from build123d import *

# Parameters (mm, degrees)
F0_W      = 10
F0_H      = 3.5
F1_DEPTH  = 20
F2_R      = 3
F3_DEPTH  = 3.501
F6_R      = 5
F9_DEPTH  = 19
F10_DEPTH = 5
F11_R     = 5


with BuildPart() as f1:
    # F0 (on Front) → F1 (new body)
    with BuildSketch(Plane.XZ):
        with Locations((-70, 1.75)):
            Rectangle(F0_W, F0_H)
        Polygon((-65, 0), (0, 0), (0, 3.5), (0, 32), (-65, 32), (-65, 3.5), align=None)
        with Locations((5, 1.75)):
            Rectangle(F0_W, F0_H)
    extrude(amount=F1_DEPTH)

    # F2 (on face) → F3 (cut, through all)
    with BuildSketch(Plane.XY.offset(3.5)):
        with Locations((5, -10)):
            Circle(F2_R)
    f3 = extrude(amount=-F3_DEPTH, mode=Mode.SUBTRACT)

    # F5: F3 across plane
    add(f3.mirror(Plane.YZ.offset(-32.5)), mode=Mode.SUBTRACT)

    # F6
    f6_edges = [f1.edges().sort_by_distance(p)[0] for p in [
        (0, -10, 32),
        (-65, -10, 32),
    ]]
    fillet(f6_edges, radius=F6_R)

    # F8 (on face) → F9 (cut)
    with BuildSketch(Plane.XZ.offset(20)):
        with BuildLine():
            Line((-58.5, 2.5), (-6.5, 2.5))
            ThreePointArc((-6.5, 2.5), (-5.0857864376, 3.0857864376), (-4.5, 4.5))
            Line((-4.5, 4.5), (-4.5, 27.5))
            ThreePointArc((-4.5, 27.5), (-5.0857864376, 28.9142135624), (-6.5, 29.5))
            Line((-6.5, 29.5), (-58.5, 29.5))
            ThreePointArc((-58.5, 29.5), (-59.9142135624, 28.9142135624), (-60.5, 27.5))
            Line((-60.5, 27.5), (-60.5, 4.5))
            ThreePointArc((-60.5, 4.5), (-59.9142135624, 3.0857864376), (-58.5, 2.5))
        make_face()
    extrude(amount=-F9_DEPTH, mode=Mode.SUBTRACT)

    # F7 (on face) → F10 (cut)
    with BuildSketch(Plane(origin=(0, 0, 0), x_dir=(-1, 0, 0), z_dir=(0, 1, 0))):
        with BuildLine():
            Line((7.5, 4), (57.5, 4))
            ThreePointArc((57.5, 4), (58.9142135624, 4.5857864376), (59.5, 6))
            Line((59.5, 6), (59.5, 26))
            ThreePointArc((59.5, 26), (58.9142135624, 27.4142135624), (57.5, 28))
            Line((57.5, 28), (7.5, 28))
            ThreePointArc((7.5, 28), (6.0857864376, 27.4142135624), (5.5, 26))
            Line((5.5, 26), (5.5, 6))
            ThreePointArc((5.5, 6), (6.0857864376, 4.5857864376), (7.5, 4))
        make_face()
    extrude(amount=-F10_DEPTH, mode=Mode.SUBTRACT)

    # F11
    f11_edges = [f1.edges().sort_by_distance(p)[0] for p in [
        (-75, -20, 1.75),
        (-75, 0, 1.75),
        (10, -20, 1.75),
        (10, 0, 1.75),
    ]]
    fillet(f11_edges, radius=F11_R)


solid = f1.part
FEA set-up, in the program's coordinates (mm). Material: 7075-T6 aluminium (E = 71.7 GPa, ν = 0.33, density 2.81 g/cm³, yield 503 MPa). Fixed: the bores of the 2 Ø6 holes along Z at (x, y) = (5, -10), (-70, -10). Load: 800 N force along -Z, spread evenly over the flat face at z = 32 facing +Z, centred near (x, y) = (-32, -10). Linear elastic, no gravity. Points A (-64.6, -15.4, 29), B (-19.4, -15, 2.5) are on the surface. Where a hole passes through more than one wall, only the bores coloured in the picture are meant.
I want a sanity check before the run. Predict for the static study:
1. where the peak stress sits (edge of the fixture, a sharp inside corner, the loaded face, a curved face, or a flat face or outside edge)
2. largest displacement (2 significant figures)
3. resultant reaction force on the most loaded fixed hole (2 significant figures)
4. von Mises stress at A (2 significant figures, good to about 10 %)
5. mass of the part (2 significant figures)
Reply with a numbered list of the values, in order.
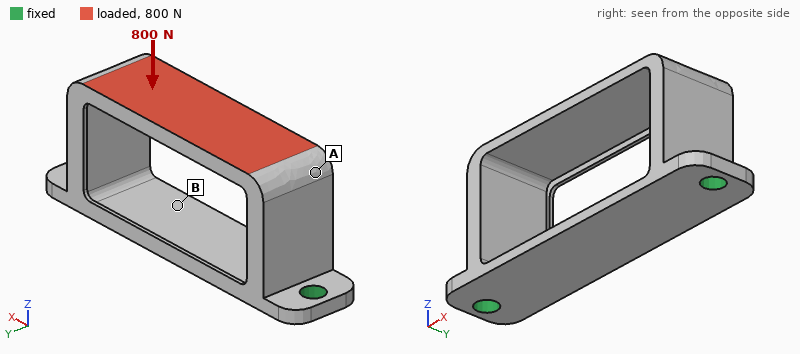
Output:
1. a curved face
2. 0.24 mm
3. 460 N
4. 35 MPa
5. 35 g
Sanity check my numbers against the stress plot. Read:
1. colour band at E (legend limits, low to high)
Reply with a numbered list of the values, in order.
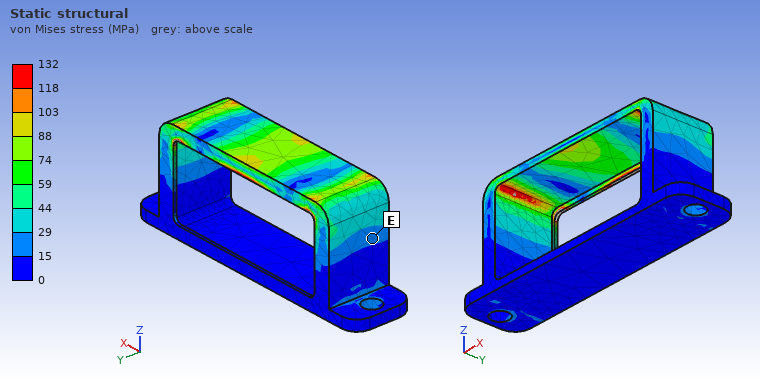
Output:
1. 15 to 29 MPa
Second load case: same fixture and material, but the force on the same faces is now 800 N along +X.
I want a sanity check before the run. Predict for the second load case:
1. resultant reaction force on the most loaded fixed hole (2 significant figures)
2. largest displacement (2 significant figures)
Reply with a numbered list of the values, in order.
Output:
1. 440 N
2. 0.32 mm
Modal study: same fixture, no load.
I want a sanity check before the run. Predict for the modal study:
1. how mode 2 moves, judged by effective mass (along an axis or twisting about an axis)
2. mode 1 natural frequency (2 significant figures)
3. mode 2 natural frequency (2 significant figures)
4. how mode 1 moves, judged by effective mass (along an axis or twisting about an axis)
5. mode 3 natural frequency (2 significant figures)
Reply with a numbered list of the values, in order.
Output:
1. along Y
2. 2200 Hz
3. 2900 Hz
4. along X
5. 3800 Hz
